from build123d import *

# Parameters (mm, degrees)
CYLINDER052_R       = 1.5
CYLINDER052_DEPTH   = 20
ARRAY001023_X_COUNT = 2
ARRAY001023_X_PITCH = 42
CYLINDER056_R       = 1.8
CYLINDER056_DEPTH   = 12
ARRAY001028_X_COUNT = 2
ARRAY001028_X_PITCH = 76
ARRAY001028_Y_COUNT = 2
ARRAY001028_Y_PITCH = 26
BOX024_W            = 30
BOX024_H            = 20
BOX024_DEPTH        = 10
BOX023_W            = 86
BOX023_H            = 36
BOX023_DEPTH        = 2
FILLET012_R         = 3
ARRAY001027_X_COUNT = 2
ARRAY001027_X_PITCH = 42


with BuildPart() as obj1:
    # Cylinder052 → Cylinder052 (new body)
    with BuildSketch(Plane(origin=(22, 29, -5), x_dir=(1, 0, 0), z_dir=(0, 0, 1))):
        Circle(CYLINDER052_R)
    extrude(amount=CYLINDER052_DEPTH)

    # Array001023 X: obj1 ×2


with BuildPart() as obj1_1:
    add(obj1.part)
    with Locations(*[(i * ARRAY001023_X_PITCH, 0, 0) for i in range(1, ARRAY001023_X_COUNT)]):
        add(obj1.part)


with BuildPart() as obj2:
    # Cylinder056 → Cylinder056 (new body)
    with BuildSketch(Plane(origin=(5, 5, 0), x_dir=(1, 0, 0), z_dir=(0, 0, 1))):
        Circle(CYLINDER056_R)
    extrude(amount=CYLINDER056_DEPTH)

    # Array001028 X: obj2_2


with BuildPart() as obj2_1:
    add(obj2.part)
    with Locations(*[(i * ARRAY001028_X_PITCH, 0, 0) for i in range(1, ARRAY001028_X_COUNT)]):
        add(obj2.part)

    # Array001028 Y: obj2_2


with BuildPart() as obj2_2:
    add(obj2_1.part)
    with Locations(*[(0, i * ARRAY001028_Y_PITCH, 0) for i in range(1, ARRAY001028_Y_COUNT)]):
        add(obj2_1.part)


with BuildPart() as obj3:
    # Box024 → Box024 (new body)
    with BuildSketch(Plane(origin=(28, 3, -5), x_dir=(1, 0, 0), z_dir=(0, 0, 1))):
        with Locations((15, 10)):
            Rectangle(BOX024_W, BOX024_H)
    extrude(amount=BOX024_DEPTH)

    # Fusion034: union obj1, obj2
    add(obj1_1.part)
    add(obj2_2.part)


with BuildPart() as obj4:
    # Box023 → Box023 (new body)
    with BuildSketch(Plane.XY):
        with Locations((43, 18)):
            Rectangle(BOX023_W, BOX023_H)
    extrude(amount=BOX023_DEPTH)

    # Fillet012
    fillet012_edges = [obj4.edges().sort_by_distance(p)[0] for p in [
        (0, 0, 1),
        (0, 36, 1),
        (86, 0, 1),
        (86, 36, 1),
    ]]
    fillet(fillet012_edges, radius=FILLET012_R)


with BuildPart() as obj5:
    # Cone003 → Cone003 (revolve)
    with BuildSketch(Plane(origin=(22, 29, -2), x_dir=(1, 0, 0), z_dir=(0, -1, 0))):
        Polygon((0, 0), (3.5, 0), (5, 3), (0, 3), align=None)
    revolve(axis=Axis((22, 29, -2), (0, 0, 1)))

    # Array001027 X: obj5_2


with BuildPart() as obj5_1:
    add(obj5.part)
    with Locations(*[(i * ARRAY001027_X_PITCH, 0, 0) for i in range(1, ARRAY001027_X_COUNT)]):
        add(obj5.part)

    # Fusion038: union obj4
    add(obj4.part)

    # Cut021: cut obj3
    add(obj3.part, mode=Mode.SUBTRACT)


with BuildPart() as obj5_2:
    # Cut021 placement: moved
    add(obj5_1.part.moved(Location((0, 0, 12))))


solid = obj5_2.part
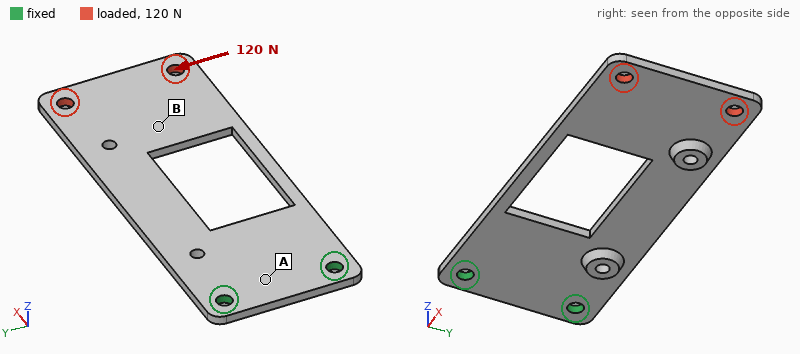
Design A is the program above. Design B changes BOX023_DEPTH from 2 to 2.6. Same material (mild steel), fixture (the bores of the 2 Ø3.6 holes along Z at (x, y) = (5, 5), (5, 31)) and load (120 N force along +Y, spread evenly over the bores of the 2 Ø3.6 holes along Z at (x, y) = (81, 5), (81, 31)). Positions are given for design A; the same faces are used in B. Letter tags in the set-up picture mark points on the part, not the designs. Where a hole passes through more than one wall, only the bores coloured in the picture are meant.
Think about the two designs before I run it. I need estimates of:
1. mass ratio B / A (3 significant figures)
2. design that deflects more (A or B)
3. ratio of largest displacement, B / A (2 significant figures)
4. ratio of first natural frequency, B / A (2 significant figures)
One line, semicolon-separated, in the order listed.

1.29; A; 0.76; 1.3
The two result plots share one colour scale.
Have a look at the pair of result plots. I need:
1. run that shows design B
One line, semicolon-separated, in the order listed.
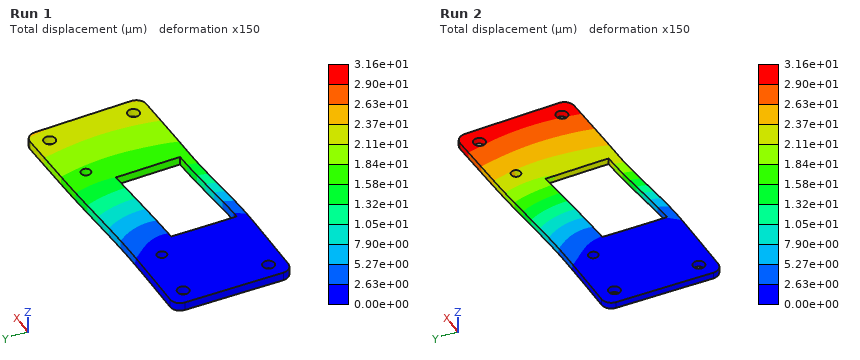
Run 1
